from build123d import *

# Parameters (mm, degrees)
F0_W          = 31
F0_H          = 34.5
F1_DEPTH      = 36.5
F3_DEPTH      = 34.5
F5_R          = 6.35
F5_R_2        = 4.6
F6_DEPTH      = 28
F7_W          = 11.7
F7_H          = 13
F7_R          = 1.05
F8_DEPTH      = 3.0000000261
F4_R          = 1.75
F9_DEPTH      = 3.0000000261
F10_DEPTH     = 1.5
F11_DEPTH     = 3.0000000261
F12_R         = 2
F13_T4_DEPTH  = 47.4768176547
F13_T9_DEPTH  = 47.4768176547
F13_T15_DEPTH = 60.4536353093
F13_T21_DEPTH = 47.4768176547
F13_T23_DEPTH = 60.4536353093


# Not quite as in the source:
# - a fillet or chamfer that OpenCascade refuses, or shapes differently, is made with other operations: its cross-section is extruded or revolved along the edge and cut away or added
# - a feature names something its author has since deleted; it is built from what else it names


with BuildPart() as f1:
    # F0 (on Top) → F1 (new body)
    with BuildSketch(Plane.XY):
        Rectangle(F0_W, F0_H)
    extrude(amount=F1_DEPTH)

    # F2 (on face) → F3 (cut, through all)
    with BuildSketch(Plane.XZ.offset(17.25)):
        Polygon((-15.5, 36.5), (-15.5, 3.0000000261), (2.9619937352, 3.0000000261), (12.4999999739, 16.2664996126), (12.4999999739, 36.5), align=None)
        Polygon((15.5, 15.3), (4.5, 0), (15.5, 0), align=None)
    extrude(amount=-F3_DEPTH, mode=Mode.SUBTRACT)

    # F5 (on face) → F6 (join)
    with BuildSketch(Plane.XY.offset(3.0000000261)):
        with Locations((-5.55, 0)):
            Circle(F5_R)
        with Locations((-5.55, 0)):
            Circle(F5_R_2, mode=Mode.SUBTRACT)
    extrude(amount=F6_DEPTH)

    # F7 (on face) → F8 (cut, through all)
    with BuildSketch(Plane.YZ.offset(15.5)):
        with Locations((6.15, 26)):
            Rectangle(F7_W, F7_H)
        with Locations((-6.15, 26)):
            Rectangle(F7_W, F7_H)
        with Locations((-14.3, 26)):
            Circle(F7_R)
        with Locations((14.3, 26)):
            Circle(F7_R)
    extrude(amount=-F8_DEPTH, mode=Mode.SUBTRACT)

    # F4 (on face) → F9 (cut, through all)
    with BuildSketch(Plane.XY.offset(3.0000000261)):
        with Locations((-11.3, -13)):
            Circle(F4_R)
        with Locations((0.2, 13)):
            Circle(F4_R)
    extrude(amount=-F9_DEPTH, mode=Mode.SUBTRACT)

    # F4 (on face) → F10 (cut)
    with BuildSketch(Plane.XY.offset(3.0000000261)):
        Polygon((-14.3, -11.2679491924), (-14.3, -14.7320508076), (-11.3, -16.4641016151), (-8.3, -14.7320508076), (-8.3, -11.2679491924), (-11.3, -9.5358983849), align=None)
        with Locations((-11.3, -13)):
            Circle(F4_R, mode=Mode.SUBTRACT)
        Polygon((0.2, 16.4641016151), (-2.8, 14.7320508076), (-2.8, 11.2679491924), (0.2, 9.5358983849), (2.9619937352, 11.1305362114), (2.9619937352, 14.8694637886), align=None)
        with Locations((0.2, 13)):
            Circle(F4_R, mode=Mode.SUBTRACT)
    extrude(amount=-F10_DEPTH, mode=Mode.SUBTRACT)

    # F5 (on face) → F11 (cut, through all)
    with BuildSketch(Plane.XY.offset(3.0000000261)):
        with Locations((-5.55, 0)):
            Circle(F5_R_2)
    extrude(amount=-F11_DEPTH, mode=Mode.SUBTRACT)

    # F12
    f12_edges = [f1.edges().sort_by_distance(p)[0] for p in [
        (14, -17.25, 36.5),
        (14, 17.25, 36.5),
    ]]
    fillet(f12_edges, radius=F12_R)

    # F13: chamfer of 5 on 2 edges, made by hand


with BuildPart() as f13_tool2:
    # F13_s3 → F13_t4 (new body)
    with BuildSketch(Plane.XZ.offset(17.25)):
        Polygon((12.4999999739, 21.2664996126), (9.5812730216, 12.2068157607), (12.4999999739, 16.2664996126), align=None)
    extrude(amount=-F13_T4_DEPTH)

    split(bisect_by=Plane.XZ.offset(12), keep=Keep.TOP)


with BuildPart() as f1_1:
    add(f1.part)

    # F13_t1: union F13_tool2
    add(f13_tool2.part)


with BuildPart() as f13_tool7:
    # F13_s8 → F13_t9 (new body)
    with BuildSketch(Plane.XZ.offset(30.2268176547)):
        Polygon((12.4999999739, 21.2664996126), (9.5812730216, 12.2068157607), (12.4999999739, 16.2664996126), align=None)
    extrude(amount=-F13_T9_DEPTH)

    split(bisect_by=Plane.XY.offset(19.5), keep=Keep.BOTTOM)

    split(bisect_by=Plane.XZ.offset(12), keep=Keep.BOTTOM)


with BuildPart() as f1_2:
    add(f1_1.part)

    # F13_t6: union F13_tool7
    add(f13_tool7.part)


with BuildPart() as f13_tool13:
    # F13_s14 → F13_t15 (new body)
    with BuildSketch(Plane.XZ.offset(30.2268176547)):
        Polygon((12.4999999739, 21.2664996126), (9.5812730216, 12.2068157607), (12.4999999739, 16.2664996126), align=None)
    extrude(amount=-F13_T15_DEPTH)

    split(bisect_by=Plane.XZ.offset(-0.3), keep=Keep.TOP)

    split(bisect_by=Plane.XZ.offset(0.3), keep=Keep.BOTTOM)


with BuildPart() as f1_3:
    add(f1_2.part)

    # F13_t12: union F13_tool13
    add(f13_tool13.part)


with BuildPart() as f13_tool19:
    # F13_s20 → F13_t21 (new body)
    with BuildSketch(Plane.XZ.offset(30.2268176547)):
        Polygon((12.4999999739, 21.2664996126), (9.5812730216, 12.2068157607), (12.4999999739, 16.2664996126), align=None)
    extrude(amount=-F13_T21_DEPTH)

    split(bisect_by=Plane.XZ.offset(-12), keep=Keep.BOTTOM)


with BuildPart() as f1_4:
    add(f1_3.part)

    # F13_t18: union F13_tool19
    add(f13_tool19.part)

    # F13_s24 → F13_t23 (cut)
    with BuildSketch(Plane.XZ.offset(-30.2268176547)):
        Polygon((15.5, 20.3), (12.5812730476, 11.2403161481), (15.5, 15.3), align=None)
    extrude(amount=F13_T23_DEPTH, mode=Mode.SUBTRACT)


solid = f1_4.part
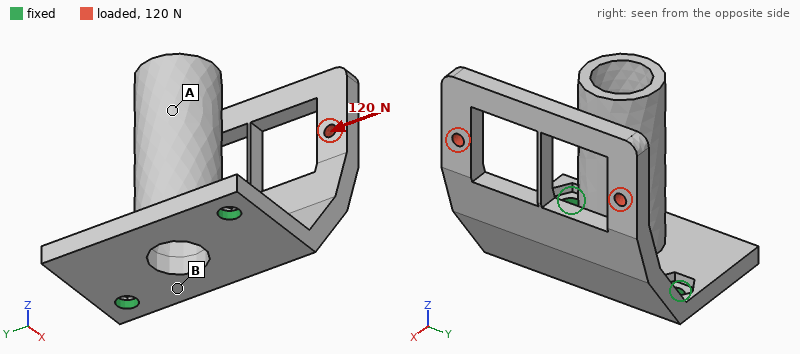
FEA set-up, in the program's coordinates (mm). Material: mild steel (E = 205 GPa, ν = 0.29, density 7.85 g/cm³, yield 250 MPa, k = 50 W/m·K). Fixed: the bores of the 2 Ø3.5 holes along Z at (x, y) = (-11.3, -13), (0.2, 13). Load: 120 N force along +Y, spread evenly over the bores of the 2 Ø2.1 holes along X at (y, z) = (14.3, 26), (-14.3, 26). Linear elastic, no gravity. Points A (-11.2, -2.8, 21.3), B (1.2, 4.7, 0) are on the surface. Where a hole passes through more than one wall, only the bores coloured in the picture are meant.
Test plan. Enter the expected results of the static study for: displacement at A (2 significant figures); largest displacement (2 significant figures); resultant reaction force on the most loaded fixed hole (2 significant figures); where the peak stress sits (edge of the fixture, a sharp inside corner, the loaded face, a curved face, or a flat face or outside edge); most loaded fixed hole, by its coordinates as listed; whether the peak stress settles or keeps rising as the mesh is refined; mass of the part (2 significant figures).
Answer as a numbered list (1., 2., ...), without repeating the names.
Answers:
1. 16 µm
2. 59 µm
3. 150 N
4. edge of the fixture
5. (-11.3, -13)
6. keeps rising
7. 50 g
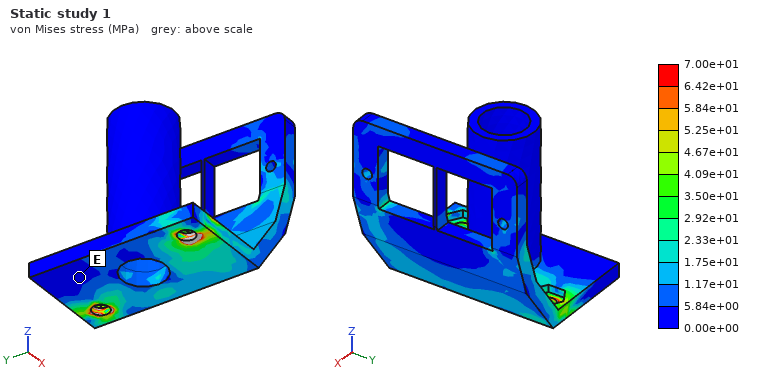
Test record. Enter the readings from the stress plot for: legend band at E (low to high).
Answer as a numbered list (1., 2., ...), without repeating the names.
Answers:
1. 0.00e+00 to 5.84e+00 MPa
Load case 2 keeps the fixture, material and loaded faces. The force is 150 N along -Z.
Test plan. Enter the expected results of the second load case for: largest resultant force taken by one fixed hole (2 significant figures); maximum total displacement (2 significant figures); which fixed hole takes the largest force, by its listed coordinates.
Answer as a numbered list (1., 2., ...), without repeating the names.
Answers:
1. 120 N
2. 0.11 mm
3. (0.2, 13)
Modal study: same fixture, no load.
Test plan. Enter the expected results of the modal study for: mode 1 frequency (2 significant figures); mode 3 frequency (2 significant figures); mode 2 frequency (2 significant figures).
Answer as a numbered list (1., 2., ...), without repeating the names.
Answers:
1. 1300 Hz
2. 3700 Hz
3. 2600 Hz
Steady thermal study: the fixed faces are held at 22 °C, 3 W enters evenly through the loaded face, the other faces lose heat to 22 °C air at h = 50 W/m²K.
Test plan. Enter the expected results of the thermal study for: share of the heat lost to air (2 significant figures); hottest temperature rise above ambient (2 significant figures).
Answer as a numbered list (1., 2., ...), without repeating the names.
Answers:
1. 57 %
2. 24 K
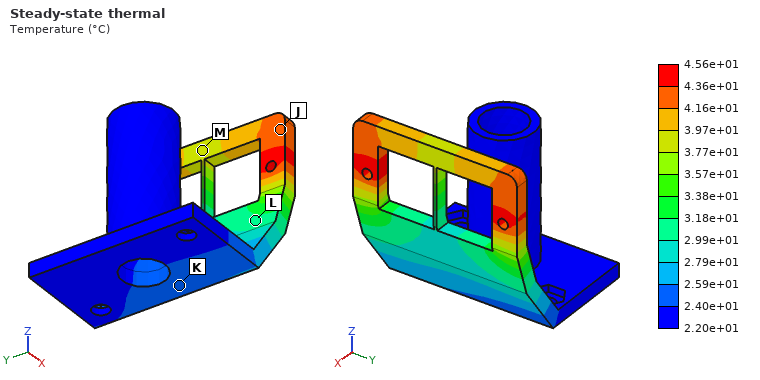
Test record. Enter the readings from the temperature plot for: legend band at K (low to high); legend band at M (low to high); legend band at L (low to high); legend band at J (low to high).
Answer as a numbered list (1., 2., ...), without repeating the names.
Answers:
1. 2.40e+01 to 2.59e+01 °C
2. 3.77e+01 to 3.97e+01 °C
3. 2.99e+01 to 3.18e+01 °C
4. 4.16e+01 to 4.36e+01 °C
